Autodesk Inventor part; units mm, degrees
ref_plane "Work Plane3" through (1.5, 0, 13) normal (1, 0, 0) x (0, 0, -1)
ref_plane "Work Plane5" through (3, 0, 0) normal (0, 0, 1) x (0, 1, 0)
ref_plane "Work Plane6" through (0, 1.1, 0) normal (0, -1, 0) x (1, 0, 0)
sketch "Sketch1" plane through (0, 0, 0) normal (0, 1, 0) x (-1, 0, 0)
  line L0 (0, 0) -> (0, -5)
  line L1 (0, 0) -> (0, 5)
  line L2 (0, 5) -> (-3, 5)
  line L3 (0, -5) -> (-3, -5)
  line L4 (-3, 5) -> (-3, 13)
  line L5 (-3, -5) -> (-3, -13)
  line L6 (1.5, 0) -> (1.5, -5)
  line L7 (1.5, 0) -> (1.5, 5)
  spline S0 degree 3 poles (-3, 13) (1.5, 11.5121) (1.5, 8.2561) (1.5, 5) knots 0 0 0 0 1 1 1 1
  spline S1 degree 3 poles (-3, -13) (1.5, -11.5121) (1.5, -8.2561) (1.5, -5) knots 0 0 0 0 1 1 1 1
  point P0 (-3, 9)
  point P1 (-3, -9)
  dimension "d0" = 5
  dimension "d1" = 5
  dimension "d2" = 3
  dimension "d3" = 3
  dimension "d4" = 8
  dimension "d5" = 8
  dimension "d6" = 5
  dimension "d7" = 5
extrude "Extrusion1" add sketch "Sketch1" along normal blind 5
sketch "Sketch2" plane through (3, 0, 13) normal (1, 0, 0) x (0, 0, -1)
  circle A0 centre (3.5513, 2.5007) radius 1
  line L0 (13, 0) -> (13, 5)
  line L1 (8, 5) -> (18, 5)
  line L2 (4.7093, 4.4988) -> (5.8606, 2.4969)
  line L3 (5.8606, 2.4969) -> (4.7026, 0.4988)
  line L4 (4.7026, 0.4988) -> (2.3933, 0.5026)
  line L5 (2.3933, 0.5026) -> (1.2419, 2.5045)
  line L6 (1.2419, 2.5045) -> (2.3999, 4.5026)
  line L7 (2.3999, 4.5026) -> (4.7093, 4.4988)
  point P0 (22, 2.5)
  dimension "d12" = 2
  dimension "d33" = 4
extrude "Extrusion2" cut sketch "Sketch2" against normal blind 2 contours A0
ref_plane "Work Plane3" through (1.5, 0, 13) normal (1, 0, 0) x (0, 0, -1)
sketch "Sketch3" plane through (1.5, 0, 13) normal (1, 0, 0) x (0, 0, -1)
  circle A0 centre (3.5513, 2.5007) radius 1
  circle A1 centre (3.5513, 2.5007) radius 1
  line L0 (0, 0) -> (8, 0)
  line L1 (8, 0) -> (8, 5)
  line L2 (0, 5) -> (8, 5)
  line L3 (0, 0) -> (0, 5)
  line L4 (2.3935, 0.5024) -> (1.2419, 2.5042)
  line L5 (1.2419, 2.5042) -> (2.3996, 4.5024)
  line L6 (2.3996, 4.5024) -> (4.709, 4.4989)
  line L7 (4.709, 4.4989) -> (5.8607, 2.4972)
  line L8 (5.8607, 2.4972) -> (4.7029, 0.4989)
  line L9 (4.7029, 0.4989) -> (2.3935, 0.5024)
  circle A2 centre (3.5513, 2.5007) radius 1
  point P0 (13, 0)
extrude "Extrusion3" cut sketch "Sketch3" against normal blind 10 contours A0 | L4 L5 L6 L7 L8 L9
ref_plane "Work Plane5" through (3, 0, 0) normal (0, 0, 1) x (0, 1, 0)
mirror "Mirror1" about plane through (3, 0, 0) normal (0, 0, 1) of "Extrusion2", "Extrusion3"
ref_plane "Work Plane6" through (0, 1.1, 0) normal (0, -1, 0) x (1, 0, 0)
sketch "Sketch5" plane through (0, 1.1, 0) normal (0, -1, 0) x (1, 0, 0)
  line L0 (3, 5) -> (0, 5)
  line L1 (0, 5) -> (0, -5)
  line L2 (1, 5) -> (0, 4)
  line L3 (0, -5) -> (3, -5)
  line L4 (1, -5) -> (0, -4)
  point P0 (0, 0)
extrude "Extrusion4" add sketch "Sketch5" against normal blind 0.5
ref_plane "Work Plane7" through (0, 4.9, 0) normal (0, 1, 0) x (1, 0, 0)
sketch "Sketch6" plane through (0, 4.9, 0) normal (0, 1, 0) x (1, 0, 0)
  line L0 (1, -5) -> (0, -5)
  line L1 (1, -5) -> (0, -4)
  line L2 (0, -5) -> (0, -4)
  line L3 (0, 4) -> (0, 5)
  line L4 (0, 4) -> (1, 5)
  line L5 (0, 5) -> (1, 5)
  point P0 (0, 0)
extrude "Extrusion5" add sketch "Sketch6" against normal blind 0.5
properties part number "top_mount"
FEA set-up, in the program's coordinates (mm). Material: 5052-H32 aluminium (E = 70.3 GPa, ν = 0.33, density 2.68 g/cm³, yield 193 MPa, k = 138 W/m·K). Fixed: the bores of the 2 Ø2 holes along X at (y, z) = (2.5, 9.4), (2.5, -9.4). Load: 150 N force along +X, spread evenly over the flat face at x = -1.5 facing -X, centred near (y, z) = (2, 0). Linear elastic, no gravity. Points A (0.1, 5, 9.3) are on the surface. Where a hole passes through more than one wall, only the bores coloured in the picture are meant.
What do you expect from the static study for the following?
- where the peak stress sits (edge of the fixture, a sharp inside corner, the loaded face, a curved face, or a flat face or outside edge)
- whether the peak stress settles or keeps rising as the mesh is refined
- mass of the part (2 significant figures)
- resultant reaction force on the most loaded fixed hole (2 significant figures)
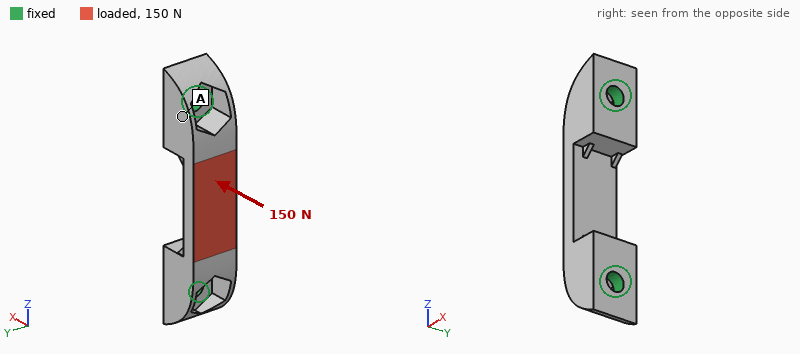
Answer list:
edge of the fixture
keeps rising
0.78 g
130 N
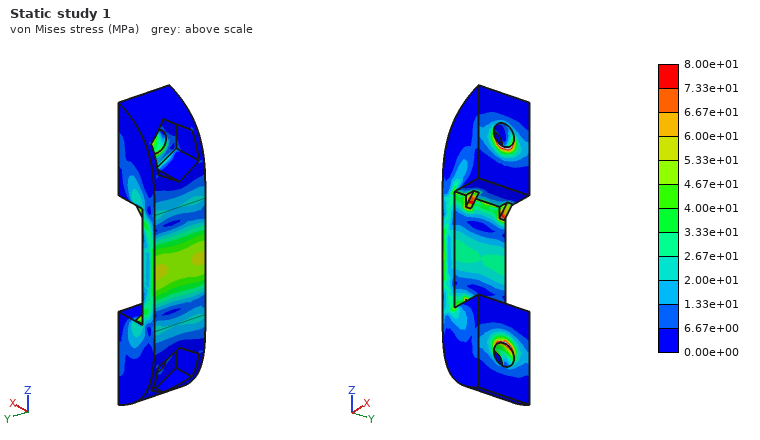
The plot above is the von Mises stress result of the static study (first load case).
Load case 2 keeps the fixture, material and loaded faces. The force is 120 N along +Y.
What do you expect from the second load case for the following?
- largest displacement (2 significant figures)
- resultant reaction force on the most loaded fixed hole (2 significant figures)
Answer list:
12 µm
60 N
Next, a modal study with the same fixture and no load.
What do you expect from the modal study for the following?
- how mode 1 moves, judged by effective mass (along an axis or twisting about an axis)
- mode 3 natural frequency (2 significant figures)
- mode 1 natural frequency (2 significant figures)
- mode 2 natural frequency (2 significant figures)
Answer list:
along Y
45 kHz
34 kHz
45 kHz
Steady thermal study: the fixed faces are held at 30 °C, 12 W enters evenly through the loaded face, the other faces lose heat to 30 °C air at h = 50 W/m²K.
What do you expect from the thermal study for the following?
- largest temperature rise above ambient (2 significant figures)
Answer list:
34 K
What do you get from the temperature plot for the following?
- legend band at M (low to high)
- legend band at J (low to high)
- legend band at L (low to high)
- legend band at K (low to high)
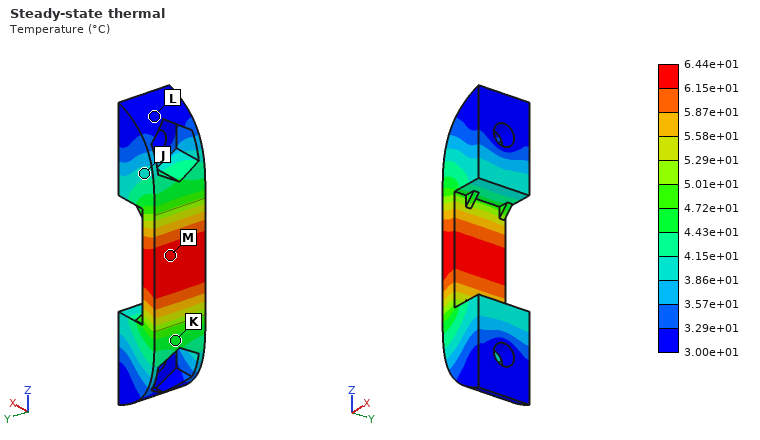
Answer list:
6.15e+01 to 6.44e+01 °C
3.86e+01 to 4.15e+01 °C
3.00e+01 to 3.29e+01 °C
4.43e+01 to 4.72e+01 °C
